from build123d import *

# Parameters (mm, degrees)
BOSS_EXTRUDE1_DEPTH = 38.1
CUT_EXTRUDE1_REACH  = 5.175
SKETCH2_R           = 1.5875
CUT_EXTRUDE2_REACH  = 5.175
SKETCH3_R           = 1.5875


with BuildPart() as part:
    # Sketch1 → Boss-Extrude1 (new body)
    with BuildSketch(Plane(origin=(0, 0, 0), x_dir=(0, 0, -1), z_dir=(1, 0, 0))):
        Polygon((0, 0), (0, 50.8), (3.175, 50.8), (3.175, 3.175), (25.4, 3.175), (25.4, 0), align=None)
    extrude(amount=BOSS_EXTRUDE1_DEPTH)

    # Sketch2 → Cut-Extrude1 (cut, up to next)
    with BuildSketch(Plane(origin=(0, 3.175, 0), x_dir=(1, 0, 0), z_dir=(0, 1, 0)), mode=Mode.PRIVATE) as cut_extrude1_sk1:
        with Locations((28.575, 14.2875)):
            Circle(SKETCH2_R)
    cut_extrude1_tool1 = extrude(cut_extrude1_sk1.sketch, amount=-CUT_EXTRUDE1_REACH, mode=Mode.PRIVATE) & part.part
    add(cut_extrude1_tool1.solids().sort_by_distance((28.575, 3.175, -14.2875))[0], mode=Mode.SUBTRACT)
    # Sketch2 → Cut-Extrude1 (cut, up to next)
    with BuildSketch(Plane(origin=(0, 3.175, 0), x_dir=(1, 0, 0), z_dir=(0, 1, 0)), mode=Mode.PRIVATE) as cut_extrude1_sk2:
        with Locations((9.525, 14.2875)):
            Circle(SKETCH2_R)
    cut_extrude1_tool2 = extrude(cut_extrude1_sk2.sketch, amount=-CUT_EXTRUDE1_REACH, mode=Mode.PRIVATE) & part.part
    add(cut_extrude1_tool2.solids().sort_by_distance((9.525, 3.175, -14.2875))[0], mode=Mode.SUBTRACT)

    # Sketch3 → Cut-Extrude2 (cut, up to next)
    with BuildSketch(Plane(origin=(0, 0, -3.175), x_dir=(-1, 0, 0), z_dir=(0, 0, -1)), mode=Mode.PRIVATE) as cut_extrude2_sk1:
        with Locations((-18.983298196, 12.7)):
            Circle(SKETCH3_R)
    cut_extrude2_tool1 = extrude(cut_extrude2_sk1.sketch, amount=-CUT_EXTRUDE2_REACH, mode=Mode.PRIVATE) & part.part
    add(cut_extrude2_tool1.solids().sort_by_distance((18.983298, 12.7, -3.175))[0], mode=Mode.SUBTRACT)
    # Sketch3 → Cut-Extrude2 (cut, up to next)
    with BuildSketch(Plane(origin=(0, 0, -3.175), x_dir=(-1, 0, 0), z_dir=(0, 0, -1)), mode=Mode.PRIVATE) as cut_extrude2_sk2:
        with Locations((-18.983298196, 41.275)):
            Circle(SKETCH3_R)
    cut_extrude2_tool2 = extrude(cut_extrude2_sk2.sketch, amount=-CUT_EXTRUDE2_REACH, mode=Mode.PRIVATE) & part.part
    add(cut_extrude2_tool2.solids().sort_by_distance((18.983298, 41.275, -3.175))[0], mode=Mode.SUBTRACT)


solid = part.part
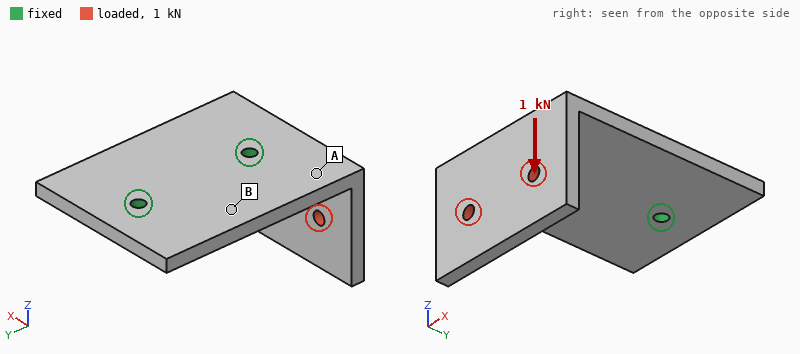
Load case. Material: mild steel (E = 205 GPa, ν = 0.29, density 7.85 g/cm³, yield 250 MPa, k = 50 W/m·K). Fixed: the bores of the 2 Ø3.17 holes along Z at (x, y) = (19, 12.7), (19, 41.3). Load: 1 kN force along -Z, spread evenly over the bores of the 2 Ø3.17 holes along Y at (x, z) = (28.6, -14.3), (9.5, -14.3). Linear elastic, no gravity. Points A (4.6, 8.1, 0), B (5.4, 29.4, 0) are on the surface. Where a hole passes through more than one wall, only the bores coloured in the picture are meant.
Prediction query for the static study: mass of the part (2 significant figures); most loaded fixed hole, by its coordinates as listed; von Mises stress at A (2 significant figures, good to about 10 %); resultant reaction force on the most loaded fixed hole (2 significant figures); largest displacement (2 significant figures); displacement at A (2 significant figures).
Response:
69 g
(19, 12.7)
61 MPa
1.1 kN
0.11 mm
0.017 mm
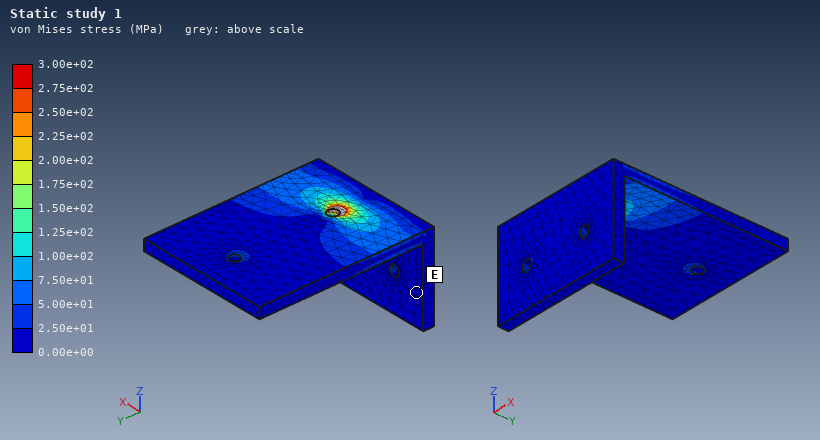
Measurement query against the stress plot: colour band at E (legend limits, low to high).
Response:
0.00e+00 to 2.50e+01 MPa
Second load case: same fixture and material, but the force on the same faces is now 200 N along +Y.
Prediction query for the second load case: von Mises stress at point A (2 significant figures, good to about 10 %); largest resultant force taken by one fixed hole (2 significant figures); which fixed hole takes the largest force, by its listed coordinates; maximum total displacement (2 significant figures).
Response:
30 MPa
160 N
(19, 12.7)
51 µm
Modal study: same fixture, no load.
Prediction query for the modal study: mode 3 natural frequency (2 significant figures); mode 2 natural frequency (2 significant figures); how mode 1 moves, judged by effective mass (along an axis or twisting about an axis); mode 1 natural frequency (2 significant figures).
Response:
6100 Hz
2800 Hz
along Y
2500 Hz
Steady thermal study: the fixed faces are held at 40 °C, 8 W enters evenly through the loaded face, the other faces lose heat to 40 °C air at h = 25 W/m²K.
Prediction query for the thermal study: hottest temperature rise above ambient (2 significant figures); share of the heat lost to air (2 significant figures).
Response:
36 K
25 %
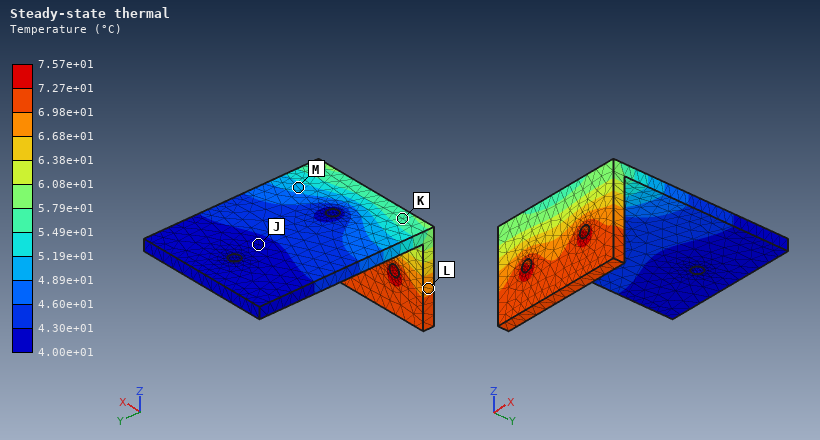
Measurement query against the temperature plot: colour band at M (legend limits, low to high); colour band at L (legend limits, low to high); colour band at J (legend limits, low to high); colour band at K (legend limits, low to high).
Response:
4.89e+01 to 5.19e+01 °C
6.68e+01 to 6.98e+01 °C
4.00e+01 to 4.30e+01 °C
5.49e+01 to 5.79e+01 °C
